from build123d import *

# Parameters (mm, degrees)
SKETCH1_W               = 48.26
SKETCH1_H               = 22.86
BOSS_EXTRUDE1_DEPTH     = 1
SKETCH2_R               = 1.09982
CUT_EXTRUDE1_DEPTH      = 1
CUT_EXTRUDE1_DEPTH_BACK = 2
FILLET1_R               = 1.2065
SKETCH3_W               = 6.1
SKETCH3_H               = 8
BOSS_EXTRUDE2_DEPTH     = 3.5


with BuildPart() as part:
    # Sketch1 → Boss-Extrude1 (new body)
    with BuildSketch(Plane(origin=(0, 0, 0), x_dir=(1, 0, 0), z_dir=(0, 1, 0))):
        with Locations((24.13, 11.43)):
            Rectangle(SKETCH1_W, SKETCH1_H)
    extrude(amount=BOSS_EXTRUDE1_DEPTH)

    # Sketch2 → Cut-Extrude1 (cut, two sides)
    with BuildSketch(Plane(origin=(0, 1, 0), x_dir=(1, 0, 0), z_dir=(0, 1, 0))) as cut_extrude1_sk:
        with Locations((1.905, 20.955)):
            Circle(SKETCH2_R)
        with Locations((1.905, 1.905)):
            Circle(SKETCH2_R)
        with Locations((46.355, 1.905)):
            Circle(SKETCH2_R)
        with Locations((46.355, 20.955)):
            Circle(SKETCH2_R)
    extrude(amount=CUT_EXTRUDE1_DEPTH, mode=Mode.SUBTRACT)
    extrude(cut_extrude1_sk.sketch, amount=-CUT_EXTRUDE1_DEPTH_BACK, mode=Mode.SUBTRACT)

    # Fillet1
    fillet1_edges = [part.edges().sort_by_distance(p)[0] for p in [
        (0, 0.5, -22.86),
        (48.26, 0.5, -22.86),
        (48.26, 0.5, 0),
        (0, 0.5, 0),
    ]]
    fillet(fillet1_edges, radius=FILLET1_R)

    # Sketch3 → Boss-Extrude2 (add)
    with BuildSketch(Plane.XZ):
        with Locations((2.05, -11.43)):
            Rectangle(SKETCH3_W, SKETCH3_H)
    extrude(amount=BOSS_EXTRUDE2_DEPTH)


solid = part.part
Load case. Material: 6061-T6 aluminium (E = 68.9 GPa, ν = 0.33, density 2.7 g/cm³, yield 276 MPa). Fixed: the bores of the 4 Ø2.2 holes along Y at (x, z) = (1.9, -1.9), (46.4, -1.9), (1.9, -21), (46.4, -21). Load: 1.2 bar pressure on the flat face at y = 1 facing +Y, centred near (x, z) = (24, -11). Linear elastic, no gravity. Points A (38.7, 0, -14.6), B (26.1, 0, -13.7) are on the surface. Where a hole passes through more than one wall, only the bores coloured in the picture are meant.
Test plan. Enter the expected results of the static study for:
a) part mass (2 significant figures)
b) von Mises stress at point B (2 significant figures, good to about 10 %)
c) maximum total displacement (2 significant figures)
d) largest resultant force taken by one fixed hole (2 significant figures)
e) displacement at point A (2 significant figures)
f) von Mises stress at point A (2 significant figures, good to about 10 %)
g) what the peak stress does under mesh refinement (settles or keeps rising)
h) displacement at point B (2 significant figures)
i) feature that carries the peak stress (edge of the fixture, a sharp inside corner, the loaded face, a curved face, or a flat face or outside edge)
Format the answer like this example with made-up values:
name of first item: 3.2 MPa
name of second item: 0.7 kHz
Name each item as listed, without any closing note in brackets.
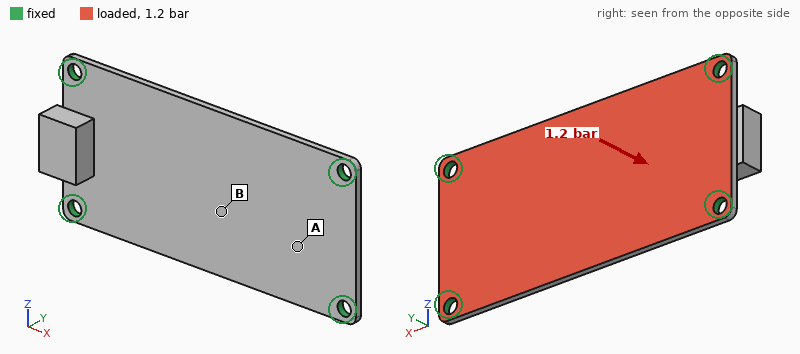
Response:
part mass: 3.4 g
von Mises stress at point B: 54 MPa
maximum total displacement: 0.24 mm
largest resultant force taken by one fixed hole: 33 N
displacement at point A: 0.090 mm
von Mises stress at point A: 18 MPa
what the peak stress does under mesh refinement: keeps rising
displacement at point B: 0.22 mm
feature that carries the peak stress: edge of the fixture
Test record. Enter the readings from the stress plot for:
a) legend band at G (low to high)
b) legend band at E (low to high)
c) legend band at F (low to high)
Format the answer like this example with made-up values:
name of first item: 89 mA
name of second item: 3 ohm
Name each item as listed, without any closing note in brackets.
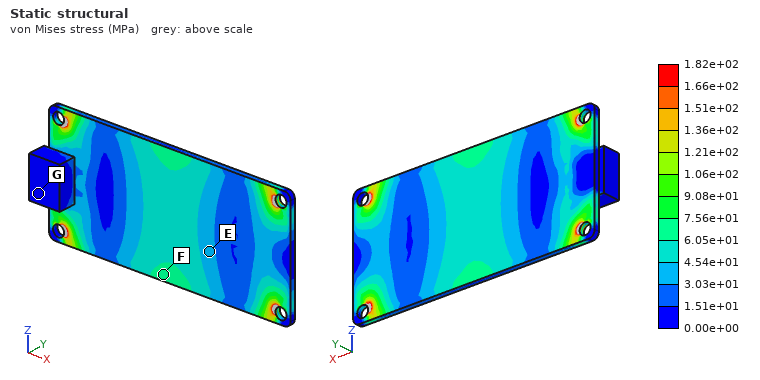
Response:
legend band at G: 0.00e+00 to 1.51e+01 MPa
legend band at E: 3.03e+01 to 4.54e+01 MPa
legend band at F: 6.05e+01 to 7.56e+01 MPa
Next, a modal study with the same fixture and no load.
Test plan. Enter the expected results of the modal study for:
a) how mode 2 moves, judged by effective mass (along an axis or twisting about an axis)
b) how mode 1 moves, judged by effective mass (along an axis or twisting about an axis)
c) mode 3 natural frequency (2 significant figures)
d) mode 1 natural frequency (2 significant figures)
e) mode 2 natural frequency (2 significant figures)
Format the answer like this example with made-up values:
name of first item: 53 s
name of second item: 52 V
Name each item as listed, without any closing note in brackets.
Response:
how mode 2 moves, judged by effective mass: twisting about X
how mode 1 moves, judged by effective mass: along Y
mode 3 natural frequency: 6900 Hz
mode 1 natural frequency: 2500 Hz
mode 2 natural frequency: 4500 Hz
